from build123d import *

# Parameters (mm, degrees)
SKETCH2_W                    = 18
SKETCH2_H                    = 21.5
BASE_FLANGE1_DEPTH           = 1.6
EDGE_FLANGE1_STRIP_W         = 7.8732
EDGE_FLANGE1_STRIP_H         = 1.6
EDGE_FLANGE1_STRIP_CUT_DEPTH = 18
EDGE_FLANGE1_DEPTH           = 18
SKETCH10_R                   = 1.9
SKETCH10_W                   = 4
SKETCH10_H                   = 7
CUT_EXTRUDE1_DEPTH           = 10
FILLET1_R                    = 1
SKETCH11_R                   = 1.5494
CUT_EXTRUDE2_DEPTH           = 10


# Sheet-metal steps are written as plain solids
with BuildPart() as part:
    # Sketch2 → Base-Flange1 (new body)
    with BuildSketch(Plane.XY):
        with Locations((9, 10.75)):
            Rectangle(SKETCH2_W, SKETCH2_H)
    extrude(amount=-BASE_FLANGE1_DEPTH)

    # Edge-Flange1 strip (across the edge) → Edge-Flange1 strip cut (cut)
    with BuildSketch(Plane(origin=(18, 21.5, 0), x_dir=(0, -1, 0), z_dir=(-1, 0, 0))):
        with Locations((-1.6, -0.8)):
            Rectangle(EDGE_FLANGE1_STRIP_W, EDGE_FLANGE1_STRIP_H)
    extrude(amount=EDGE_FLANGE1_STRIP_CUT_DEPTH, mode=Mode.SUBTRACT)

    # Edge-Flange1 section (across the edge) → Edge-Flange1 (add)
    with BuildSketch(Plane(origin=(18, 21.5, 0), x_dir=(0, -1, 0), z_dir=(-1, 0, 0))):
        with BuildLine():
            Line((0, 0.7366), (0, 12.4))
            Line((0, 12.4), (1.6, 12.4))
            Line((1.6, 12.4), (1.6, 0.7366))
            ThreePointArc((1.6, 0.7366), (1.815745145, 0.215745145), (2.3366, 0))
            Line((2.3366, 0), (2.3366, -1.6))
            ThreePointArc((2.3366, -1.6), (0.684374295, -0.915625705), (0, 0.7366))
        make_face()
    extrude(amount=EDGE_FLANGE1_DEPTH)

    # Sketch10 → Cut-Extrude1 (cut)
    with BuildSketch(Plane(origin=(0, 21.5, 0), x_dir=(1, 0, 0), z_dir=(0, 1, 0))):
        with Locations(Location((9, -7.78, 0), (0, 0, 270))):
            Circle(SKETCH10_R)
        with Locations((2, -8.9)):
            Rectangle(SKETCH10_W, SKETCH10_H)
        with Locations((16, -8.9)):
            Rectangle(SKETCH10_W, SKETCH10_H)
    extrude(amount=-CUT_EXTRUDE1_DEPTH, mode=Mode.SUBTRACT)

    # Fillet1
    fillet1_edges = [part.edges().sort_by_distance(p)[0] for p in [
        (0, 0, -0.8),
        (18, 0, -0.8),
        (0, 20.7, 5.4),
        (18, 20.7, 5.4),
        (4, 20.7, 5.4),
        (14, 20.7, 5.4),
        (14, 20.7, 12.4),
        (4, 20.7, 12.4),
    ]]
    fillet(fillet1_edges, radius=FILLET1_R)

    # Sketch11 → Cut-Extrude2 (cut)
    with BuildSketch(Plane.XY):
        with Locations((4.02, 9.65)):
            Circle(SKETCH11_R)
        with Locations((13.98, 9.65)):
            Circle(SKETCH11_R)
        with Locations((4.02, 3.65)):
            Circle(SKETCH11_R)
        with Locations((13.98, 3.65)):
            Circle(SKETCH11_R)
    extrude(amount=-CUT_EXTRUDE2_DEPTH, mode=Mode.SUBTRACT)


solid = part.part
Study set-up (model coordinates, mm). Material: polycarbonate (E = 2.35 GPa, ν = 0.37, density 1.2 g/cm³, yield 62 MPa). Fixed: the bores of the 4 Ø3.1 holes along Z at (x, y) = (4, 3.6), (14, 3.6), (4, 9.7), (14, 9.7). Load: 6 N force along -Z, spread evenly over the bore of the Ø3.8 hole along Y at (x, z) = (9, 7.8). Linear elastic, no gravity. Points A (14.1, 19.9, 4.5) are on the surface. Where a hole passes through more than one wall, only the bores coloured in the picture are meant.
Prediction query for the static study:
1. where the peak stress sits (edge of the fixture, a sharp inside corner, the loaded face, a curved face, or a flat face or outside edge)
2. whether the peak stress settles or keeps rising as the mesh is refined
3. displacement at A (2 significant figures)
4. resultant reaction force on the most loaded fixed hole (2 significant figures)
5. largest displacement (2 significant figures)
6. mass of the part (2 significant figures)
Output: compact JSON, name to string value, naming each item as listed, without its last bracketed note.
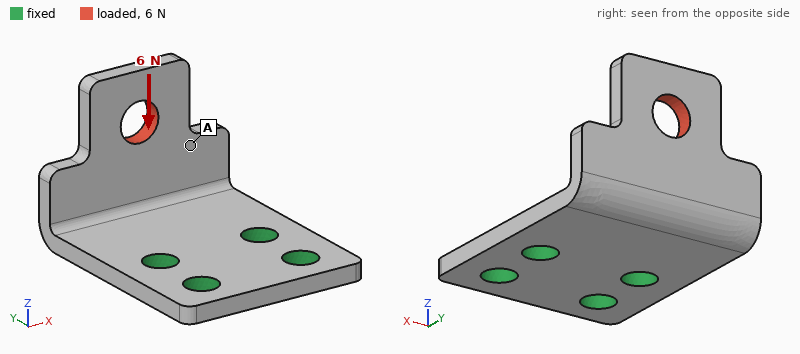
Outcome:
{"where the peak stress sits": "edge of the fixture", "whether the peak stress settles or keeps rising as the mesh is refined": "keeps rising", "displacement at A": "0.16 mm", "resultant reaction force on the most loaded fixed hole": "3.6 N", "largest displacement": "0.30 mm", "mass of the part": "0.96 g"}
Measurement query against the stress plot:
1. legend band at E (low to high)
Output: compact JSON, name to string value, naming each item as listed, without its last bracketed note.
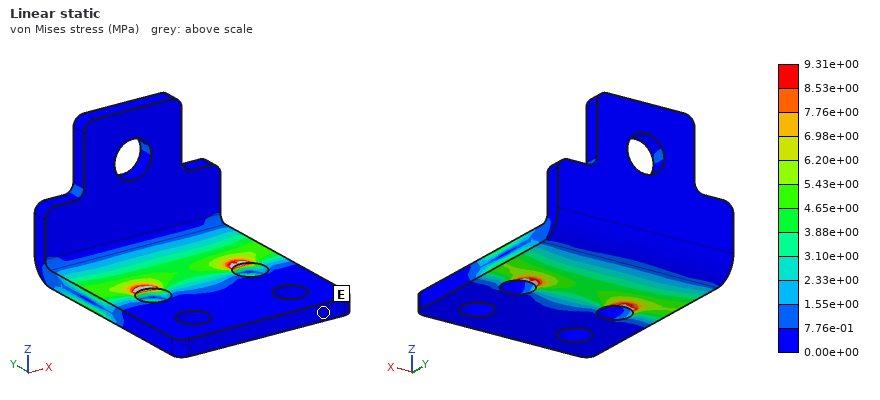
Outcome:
{"legend band at E": "0.00e+00 to 7.76e-01 MPa"}
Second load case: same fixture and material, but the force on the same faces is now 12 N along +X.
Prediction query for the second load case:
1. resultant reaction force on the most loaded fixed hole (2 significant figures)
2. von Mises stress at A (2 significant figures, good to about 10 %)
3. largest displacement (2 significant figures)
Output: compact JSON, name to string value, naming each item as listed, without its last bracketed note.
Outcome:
{"resultant reaction force on the most loaded fixed hole": "14 N", "von Mises stress at A": "4.7 MPa", "largest displacement": "0.35 mm"}
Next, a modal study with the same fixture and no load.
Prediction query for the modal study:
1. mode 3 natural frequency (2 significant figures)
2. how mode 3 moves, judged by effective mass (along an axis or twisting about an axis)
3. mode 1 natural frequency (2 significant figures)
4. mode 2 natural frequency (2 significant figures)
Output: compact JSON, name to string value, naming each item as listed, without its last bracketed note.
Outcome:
{"mode 3 natural frequency": "3000 Hz", "how mode 3 moves, judged by effective mass": "along Z", "mode 1 natural frequency": "1200 Hz", "mode 2 natural frequency": "2100 Hz"}
